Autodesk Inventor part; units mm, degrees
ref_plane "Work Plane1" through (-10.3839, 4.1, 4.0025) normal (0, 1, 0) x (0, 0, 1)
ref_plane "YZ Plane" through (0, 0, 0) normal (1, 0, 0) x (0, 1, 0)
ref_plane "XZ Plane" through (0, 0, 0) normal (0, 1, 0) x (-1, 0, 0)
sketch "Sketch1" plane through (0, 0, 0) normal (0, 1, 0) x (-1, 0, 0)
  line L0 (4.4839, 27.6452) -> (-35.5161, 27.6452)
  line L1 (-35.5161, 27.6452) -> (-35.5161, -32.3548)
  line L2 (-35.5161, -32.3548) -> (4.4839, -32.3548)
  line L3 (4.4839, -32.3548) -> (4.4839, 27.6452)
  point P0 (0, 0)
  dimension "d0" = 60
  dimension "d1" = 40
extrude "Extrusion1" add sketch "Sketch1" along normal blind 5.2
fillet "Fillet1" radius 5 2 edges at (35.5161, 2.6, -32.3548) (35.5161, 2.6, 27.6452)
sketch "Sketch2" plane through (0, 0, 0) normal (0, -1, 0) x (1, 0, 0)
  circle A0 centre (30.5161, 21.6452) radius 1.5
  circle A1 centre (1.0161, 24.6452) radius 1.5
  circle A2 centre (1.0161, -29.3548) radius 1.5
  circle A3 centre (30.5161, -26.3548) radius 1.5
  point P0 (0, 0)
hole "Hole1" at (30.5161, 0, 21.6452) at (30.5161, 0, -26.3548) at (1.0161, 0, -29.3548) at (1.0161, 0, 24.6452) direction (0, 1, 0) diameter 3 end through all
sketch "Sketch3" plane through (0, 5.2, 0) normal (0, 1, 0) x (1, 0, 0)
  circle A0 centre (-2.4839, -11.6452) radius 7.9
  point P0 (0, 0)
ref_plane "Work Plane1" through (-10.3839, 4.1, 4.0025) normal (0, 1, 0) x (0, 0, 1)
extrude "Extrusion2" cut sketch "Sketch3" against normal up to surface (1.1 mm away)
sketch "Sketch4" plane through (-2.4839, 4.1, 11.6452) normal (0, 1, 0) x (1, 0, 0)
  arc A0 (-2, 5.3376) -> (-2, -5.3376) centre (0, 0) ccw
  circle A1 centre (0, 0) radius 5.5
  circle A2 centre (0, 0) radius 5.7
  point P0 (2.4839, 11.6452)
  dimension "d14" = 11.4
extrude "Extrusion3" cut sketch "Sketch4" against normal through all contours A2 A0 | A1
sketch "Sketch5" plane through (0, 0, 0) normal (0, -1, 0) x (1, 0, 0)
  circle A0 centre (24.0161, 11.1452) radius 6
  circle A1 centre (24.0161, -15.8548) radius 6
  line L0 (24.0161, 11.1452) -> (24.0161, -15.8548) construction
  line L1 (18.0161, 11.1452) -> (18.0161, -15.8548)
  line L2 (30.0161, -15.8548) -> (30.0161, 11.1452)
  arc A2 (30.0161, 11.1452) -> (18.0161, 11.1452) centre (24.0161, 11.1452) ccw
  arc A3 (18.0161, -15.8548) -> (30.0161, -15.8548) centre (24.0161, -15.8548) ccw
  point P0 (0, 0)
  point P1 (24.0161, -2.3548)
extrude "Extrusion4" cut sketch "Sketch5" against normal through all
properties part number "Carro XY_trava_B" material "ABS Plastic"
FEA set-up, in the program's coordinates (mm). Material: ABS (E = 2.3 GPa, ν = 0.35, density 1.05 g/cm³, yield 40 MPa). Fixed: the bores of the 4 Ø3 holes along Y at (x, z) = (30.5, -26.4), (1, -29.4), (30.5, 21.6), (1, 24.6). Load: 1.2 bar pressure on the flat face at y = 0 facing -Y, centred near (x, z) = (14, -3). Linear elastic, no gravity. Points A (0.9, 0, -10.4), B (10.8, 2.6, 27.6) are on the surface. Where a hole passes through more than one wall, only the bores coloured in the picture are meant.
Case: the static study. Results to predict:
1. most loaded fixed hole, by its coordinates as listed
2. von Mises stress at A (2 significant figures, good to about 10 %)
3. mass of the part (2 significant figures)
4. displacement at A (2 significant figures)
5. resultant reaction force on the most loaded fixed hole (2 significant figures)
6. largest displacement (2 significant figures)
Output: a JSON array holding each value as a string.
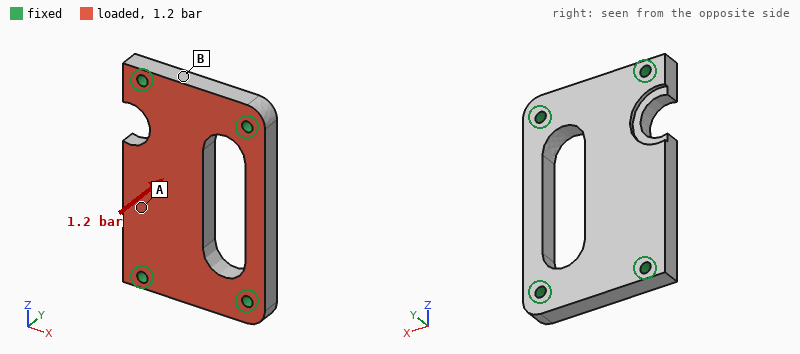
["(1, -29.4)", "2.5 MPa", "10 g", "0.12 mm", "66 N", "0.16 mm"]
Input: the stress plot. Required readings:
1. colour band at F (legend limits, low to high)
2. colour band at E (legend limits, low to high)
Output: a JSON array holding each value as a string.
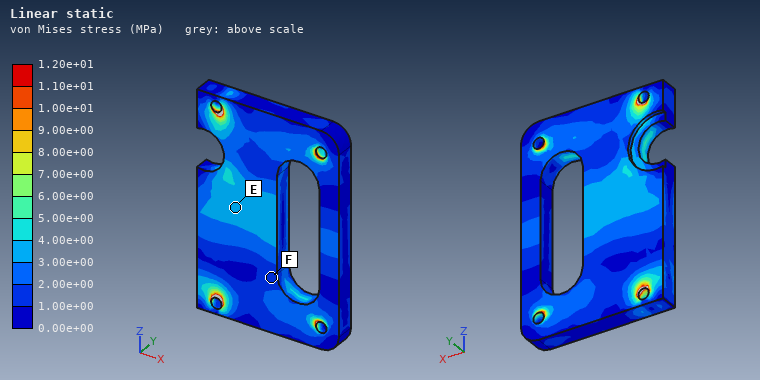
["1.00e+00 to 2.00e+00 MPa", "3.00e+00 to 4.00e+00 MPa"]
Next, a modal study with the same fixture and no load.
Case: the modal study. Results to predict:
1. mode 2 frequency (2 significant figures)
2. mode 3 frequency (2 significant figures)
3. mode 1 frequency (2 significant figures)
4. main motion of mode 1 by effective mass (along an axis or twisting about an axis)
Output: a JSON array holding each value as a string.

["3700 Hz", "4100 Hz", "2200 Hz", "along Y"]
